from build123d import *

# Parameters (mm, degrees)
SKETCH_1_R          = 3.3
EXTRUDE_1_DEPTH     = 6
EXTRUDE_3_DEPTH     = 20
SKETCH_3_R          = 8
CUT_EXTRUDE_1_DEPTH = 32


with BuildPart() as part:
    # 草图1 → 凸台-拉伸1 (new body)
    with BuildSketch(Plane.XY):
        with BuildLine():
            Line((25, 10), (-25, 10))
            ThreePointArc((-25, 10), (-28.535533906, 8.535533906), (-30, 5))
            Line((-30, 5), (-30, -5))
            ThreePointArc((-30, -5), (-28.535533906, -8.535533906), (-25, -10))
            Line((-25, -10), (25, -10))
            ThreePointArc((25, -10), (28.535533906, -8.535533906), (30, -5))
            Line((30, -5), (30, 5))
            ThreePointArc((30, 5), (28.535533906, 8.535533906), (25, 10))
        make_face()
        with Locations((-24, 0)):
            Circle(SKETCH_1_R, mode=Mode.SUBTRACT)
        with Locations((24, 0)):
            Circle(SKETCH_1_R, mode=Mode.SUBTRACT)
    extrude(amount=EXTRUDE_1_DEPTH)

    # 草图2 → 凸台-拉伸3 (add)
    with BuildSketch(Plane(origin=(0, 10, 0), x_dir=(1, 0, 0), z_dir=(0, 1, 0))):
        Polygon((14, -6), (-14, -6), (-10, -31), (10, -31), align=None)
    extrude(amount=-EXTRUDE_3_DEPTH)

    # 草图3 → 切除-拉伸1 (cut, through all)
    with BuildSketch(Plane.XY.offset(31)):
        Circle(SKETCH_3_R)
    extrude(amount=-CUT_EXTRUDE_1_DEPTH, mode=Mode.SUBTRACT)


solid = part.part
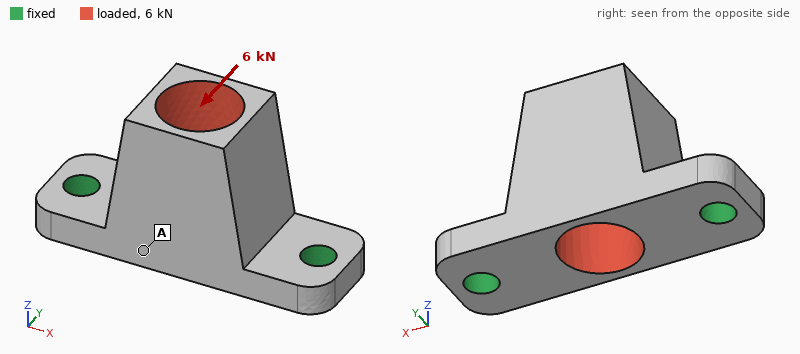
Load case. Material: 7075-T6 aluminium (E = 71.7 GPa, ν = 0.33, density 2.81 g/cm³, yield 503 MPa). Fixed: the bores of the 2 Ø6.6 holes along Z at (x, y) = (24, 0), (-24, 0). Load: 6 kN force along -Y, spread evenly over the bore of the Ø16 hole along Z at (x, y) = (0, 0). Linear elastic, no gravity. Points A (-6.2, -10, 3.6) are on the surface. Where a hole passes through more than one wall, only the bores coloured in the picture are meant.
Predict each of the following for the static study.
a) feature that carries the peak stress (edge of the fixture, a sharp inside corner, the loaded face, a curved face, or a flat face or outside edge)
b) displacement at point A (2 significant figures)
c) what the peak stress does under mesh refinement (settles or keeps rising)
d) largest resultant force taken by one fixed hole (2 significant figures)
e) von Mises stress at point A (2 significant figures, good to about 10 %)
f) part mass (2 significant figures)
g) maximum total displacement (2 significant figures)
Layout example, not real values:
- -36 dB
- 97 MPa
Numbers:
- edge of the fixture
- 0.10 mm
- keeps rising
- 3.0 kN
- 64 MPa
- 35 g
- 0.34 mm
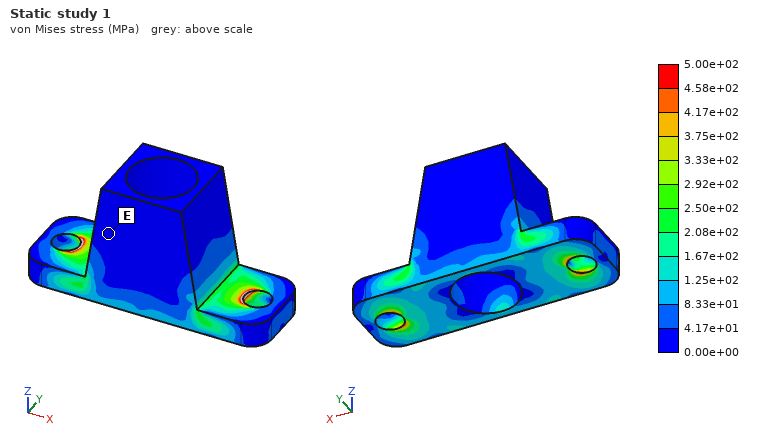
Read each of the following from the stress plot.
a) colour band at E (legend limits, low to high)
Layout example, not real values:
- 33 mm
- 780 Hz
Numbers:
- 0.00e+00 to 4.17e+01 MPa
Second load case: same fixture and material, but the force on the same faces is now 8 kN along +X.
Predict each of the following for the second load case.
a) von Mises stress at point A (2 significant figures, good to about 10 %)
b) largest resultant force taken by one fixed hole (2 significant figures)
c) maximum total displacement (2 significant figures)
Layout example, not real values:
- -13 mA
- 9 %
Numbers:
- 21 MPa
- 4.8 kN
- 70 µm
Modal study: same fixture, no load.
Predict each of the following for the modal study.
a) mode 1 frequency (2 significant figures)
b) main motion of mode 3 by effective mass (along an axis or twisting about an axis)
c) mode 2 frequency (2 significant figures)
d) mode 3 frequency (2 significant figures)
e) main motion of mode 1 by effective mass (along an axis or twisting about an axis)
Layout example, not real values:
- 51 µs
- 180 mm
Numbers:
- 5300 Hz
- along X
- 13 kHz
- 13 kHz
- along Y
